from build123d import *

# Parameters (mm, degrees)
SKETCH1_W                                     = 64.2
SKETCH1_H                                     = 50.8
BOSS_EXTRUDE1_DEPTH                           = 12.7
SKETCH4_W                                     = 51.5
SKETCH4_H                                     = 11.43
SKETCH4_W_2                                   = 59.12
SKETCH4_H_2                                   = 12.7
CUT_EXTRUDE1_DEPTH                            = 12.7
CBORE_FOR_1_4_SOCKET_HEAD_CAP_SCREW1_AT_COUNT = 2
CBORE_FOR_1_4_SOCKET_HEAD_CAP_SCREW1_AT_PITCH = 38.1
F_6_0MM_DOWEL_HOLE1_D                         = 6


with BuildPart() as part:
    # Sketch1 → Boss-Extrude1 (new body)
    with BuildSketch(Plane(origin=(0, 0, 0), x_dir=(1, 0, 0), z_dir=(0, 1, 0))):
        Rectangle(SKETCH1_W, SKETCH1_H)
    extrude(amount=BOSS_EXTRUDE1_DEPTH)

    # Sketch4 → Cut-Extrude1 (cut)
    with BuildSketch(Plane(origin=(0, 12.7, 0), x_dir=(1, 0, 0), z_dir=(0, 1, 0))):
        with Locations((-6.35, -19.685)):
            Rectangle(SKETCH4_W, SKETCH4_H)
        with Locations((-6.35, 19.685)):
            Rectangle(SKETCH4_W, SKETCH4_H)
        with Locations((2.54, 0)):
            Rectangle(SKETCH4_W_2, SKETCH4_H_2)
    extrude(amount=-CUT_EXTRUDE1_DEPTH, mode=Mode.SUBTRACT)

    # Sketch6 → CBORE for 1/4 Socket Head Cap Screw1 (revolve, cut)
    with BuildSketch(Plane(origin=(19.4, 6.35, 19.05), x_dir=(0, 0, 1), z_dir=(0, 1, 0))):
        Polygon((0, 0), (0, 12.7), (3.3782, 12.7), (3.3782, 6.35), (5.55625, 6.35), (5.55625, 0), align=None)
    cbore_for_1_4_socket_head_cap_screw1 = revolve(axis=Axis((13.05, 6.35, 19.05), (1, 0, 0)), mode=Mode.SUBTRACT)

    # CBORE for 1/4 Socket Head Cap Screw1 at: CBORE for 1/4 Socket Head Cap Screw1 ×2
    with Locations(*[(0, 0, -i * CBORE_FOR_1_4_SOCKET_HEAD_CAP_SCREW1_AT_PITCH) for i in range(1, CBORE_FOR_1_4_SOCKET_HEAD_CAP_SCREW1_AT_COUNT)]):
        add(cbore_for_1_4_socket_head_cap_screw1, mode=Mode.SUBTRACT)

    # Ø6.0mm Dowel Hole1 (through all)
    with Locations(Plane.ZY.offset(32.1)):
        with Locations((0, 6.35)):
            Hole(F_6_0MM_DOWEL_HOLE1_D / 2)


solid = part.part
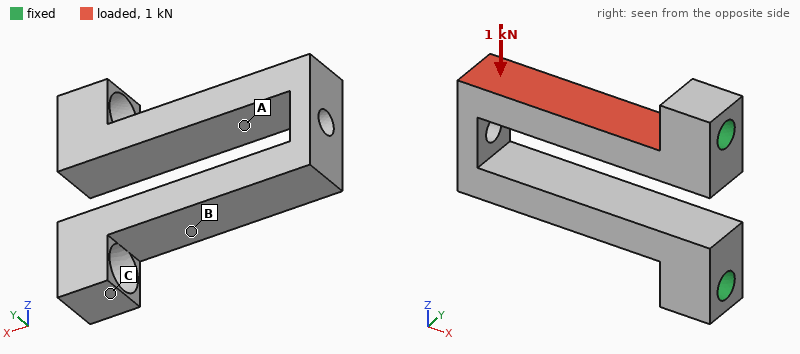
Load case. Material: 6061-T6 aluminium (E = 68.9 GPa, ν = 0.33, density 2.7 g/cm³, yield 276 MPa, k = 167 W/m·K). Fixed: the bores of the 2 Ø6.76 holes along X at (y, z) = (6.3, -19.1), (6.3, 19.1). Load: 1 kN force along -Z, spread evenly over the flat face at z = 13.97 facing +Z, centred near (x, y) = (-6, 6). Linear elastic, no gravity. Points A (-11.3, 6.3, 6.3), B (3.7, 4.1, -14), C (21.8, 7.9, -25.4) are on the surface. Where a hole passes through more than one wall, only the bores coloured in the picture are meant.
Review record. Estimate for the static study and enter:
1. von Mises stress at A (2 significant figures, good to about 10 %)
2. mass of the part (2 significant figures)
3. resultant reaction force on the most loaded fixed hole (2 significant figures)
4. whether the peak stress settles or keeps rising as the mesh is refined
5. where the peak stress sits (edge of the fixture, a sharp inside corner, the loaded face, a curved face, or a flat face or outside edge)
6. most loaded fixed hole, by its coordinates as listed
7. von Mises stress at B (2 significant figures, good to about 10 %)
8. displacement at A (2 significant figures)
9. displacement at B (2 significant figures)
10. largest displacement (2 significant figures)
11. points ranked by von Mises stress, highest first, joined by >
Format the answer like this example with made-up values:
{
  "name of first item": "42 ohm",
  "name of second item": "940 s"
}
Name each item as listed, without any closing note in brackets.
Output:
{
  "von Mises stress at A": "49 MPa",
  "mass of the part": "41 g",
  "resultant reaction force on the most loaded fixed hole": "920 N",
  "whether the peak stress settles or keeps rising as the mesh is refined": "keeps rising",
  "where the peak stress sits": "a sharp inside corner",
  "most loaded fixed hole, by its coordinates as listed": "(6.3, 19.1)",
  "von Mises stress at B": "24 MPa",
  "displacement at A": "0.16 mm",
  "displacement at B": "0.064 mm",
  "largest displacement": "0.20 mm",
  "points ranked by von Mises stress, highest first, joined by >": "A > B > C"
}
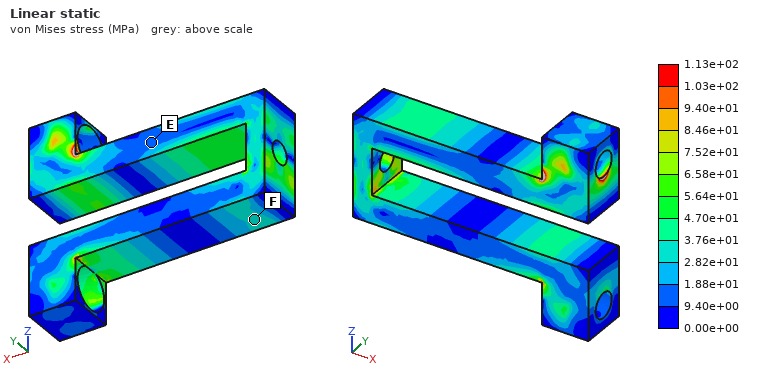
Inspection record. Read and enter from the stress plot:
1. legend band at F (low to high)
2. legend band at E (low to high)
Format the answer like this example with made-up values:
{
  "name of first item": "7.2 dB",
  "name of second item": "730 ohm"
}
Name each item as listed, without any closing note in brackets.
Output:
{
  "legend band at F": "2.82e+01 to 3.76e+01 MPa",
  "legend band at E": "9.40e+00 to 1.88e+01 MPa"
}
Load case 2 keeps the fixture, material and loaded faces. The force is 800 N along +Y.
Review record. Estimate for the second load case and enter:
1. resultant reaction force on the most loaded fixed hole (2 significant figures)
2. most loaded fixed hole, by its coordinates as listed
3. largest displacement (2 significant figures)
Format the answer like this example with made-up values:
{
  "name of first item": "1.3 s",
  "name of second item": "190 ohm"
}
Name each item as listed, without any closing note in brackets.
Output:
{
  "resultant reaction force on the most loaded fixed hole": "640 N",
  "most loaded fixed hole, by its coordinates as listed": "(6.3, 19.1)",
  "largest displacement": "0.31 mm"
}
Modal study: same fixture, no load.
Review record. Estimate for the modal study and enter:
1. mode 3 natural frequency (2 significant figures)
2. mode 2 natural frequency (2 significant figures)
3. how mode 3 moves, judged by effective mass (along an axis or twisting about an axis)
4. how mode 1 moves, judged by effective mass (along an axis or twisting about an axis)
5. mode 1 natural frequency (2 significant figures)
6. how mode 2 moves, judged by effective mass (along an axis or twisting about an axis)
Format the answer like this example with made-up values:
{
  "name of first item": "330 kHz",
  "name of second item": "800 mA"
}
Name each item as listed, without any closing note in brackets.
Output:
{
  "mode 3 natural frequency": "4700 Hz",
  "mode 2 natural frequency": "2400 Hz",
  "how mode 3 moves, judged by effective mass": "twisting about X",
  "how mode 1 moves, judged by effective mass": "along Y",
  "mode 1 natural frequency": "2000 Hz",
  "how mode 2 moves, judged by effective mass": "along Z"
}
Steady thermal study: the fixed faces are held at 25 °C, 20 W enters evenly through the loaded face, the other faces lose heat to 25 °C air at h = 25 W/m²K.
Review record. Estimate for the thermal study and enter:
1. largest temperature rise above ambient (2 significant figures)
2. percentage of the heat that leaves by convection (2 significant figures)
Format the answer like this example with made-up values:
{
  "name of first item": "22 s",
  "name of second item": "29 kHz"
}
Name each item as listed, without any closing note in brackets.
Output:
{
  "largest temperature rise above ambient": "27 K",
  "percentage of the heat that leaves by convection": "8.7 %"
}
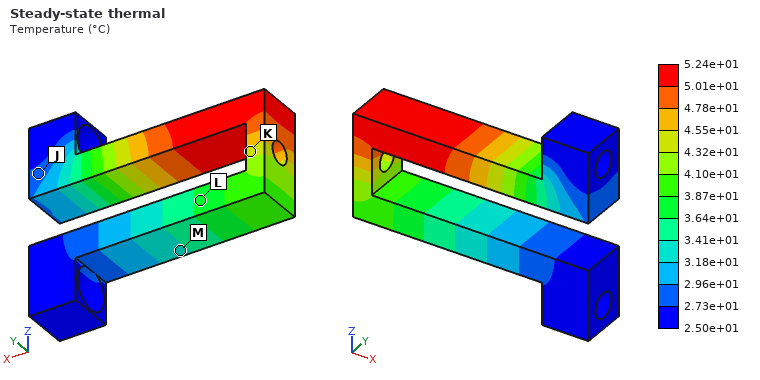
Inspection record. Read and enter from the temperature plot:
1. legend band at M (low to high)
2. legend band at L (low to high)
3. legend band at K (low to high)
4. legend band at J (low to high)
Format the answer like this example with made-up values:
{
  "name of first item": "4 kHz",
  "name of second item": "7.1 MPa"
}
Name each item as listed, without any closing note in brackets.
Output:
{
  "legend band at M": "3.18e+01 to 3.41e+01 °C",
  "legend band at L": "3.64e+01 to 3.87e+01 °C",
  "legend band at K": "4.32e+01 to 4.55e+01 °C",
  "legend band at J": "2.73e+01 to 2.96e+01 °C"
}
